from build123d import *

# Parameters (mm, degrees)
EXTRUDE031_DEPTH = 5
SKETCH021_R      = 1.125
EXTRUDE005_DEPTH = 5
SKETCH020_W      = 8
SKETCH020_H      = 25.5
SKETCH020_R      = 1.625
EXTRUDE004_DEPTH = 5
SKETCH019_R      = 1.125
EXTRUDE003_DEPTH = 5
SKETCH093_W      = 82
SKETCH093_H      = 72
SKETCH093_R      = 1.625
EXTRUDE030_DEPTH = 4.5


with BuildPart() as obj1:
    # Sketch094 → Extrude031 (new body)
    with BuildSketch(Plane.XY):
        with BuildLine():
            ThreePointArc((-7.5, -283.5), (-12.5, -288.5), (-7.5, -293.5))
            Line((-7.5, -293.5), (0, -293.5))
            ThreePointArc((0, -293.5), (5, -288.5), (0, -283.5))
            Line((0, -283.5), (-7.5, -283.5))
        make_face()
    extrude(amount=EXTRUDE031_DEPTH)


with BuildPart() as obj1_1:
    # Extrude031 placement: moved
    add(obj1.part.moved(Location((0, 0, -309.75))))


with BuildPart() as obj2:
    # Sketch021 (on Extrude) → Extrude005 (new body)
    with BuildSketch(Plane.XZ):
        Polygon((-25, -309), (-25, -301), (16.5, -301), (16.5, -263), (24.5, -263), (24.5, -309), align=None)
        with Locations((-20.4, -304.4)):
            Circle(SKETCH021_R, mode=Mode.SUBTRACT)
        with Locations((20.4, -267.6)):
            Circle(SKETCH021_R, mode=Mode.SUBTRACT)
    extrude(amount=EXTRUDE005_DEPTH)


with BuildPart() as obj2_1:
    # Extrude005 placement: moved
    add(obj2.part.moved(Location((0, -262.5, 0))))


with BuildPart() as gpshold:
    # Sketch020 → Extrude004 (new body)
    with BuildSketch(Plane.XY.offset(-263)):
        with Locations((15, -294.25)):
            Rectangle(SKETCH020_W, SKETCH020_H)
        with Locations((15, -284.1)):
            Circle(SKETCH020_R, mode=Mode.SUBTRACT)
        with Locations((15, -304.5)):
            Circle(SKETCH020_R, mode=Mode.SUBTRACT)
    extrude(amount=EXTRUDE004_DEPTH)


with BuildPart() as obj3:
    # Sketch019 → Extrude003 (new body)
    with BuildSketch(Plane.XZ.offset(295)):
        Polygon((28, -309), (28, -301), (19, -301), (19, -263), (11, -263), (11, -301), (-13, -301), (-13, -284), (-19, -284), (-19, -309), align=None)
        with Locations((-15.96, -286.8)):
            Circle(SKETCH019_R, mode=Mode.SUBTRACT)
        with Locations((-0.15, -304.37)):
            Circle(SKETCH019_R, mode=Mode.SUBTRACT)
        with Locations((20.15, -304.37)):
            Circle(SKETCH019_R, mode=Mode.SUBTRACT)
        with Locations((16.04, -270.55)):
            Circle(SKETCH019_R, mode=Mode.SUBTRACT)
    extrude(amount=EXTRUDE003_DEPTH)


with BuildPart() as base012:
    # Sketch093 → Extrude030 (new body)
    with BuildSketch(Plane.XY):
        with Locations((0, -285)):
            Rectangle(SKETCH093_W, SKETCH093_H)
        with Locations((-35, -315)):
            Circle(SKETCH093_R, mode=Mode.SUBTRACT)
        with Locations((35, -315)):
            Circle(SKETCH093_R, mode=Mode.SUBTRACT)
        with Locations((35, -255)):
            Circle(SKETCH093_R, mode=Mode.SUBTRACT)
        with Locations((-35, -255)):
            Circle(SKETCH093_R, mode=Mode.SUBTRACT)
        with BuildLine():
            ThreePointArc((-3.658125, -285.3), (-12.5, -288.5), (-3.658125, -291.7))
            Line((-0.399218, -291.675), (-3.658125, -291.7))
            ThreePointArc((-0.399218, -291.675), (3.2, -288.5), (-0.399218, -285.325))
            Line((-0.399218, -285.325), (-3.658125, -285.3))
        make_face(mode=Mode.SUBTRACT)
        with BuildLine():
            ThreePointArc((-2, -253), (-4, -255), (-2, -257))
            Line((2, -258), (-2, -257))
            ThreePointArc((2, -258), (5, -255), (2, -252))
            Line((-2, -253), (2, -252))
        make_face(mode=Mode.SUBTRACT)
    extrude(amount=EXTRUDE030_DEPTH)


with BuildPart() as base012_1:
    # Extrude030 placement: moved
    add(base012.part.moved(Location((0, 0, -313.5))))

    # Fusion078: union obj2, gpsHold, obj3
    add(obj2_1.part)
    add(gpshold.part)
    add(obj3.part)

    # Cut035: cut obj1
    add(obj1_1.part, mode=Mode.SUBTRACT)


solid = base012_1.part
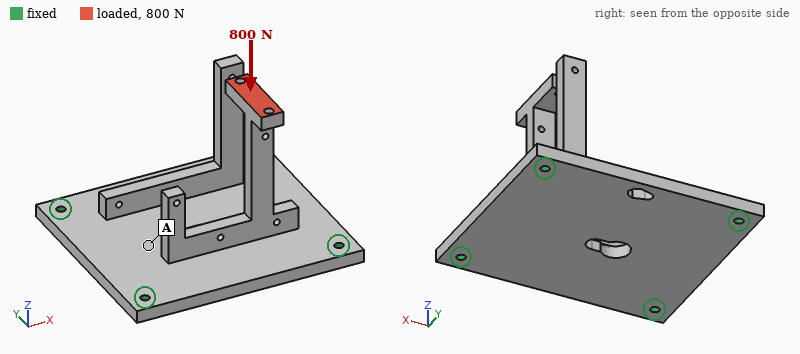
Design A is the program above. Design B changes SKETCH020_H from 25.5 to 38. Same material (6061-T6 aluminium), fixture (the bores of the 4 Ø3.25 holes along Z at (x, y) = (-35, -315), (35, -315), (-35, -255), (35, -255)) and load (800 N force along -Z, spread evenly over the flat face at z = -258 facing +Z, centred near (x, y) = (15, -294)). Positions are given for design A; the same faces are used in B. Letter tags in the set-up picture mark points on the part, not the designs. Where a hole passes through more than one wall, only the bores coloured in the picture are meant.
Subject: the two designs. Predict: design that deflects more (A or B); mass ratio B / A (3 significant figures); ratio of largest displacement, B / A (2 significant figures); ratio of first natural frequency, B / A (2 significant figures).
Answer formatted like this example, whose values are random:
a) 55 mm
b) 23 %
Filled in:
a) B
b) 1.01
c) 1.2
d) 0.83
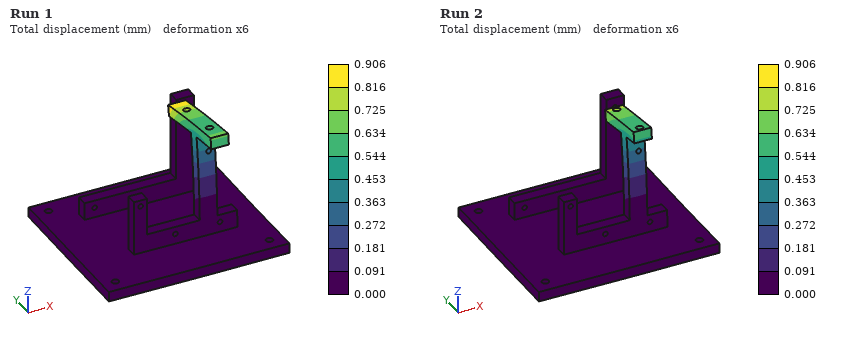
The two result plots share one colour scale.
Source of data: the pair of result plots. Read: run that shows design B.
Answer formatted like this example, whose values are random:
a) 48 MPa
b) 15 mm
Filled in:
a) Run 1
